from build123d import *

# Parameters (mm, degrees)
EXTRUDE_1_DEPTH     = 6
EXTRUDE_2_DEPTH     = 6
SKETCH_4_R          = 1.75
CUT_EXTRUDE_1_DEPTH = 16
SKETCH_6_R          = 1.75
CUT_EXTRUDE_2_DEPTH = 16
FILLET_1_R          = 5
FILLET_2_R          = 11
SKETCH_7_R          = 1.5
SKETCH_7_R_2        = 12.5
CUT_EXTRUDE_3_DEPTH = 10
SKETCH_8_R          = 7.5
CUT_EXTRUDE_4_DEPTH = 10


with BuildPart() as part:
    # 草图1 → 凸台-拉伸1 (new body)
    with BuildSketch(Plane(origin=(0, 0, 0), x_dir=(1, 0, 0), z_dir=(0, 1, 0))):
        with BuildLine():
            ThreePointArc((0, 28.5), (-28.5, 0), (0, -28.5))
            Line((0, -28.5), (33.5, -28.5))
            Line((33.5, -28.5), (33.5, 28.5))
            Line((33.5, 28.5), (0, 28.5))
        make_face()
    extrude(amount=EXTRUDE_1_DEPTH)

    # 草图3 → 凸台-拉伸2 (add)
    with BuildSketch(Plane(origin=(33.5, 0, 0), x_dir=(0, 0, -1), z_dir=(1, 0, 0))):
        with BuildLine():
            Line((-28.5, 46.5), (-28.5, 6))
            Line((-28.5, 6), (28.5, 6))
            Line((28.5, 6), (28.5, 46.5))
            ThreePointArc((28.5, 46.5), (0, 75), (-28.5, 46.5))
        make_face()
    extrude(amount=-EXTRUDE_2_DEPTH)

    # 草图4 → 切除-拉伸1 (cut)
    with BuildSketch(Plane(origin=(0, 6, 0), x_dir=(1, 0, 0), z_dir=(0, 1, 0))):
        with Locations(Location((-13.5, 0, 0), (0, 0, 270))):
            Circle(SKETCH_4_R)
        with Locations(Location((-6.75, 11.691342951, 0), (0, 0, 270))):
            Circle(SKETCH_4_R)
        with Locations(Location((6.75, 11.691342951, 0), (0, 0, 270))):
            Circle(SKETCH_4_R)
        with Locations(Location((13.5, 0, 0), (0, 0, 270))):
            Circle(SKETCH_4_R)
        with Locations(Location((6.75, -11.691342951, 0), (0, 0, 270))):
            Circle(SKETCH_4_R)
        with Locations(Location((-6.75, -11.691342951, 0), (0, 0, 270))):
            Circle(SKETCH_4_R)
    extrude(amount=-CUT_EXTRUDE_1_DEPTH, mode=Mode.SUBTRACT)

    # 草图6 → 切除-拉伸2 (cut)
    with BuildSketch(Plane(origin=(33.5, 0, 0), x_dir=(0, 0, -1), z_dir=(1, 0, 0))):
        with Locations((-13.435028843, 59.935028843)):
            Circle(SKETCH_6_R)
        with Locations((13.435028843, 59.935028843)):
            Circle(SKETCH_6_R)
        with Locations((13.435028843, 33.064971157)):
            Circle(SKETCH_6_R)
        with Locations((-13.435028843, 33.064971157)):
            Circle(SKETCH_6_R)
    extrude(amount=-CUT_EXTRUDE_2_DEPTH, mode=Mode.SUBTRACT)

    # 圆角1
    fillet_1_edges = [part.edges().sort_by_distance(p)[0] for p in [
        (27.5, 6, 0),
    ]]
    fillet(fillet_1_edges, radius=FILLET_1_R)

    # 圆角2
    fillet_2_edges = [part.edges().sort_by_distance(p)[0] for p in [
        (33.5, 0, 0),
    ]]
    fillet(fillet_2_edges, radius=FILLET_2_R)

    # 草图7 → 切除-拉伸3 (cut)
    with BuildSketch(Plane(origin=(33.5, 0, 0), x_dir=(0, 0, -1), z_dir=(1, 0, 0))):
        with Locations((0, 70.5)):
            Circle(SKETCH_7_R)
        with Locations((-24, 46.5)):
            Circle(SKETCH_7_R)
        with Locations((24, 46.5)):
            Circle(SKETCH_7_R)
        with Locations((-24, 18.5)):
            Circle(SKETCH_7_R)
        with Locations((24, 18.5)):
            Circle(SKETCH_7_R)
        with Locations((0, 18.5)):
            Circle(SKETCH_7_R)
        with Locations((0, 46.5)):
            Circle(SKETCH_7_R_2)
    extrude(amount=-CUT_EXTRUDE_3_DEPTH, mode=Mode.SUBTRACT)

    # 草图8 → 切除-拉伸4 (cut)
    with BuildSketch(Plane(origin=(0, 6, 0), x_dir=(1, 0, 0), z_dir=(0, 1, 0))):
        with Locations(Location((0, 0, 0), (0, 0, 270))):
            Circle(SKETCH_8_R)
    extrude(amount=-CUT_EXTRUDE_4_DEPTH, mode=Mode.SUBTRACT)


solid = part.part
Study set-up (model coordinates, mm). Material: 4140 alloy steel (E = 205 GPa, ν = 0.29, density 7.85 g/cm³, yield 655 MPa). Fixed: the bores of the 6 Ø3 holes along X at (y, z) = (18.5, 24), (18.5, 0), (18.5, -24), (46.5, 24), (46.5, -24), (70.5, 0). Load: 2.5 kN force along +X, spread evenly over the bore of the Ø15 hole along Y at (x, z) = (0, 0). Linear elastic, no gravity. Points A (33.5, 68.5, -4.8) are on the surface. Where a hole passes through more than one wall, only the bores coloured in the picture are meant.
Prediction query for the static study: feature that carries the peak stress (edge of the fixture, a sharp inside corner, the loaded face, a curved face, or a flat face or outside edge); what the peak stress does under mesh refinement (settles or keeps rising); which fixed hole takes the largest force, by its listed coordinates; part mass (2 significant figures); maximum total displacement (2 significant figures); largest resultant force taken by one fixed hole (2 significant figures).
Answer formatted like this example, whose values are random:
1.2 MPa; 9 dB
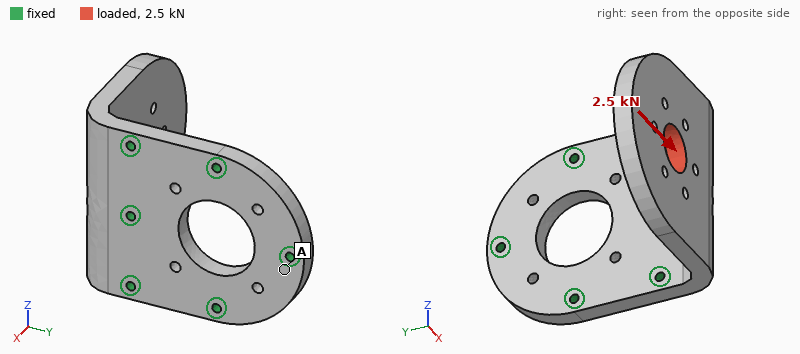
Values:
edge of the fixture; keeps rising; (18.5, 0); 270 g; 0.11 mm; 1.1 kN
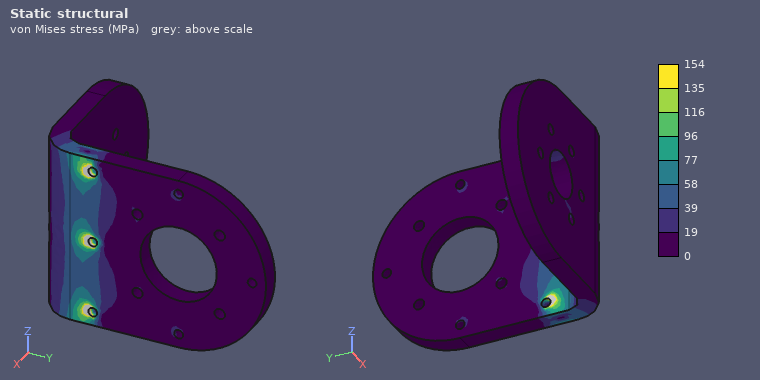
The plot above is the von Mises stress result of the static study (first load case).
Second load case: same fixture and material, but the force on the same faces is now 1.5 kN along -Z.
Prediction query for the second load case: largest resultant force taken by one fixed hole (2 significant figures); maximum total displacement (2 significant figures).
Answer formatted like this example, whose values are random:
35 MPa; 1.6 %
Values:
1.2 kN; 36 µm
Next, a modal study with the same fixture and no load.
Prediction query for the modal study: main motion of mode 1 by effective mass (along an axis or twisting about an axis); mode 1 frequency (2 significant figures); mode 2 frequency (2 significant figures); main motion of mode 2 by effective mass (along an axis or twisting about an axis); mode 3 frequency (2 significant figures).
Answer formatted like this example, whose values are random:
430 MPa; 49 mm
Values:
along Y; 1200 Hz; 3100 Hz; along Z; 4800 Hz
